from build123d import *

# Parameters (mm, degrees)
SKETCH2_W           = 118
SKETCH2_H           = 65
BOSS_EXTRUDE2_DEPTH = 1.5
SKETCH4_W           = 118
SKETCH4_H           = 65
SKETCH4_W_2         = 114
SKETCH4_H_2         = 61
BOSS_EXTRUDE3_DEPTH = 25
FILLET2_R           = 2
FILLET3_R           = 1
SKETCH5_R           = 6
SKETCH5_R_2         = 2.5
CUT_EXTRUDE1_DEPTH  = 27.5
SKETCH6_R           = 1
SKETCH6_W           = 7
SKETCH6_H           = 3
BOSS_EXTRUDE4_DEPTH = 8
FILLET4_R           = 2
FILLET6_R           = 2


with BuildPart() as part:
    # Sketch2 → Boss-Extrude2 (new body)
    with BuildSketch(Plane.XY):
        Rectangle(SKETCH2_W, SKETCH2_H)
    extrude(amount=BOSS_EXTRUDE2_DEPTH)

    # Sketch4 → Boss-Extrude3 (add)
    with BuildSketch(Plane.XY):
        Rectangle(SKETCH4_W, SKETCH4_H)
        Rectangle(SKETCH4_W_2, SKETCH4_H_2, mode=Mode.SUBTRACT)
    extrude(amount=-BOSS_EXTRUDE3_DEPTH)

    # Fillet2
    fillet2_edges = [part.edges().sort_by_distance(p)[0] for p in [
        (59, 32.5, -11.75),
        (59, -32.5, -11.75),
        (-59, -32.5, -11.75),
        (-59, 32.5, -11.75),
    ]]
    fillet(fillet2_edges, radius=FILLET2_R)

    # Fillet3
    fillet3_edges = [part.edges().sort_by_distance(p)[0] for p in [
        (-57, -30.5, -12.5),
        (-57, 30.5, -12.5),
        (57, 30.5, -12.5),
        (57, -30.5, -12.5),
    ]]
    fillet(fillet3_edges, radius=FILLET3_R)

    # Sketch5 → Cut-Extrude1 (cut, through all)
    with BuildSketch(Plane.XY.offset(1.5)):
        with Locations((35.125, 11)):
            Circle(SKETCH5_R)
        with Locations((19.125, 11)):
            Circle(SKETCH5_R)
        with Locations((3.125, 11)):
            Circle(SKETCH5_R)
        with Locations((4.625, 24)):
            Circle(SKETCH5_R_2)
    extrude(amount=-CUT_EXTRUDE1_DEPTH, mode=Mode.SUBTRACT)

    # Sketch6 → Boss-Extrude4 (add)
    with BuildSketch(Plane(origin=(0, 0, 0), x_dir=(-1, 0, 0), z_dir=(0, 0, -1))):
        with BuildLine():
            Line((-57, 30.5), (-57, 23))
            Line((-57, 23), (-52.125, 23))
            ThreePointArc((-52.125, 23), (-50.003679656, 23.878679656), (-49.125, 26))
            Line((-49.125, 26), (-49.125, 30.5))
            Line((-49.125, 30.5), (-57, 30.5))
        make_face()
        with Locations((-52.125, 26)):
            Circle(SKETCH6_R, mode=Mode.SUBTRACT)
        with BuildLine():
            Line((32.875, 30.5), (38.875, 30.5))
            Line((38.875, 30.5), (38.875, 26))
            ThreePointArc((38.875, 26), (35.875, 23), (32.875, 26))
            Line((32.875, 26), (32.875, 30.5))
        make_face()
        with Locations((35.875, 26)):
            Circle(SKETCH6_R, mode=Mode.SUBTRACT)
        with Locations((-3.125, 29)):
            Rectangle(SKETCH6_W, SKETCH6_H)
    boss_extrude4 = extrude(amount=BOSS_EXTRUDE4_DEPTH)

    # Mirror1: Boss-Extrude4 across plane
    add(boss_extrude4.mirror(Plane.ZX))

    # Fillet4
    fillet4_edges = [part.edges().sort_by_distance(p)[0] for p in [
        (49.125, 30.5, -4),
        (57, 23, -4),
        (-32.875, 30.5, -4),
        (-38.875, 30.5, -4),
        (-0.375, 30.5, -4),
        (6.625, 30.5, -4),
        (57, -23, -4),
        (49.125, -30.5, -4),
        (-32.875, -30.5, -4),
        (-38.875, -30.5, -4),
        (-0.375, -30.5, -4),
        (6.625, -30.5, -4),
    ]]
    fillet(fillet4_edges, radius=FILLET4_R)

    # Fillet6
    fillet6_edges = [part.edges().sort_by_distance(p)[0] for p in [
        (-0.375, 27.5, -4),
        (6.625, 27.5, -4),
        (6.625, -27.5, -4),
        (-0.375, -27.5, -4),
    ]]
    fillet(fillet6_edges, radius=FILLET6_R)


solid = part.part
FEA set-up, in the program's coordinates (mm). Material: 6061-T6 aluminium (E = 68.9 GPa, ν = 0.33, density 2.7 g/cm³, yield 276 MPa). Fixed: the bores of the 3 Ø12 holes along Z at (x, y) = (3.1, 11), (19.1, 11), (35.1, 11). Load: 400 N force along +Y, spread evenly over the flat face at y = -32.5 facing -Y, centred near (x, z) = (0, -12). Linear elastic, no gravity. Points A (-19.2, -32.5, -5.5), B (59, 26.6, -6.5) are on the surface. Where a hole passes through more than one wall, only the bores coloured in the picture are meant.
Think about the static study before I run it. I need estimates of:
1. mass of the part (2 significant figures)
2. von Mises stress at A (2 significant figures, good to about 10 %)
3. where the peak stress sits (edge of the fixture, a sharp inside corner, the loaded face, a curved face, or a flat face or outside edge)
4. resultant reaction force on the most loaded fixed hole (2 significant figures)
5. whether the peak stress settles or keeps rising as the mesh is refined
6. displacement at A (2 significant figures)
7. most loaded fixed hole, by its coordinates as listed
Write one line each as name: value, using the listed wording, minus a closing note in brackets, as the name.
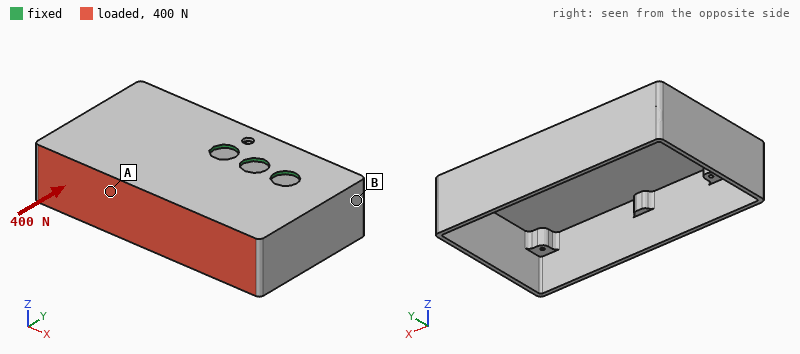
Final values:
mass of the part: 83 g
von Mises stress at A: 20 MPa
where the peak stress sits: a sharp inside corner
resultant reaction force on the most loaded fixed hole: 370 N
whether the peak stress settles or keeps rising as the mesh is refined: keeps rising
displacement at A: 0.78 mm
most loaded fixed hole, by its coordinates as listed: (3.1, 11)
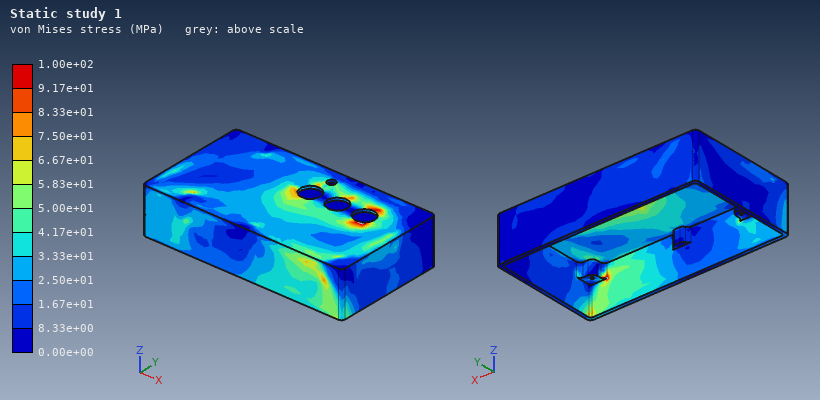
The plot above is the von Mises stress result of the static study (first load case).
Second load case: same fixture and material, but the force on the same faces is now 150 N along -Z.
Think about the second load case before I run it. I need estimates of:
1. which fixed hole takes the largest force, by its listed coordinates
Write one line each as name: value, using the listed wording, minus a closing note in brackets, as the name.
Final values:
which fixed hole takes the largest force, by its listed coordinates: (3.1, 11)
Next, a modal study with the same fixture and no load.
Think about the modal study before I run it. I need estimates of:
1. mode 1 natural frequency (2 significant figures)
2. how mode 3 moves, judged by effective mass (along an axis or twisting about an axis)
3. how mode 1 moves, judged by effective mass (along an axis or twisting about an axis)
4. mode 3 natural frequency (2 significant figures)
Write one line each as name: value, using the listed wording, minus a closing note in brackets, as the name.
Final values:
mode 1 natural frequency: 320 Hz
how mode 3 moves, judged by effective mass: along Z
how mode 1 moves, judged by effective mass: along Z
mode 3 natural frequency: 660 Hz
